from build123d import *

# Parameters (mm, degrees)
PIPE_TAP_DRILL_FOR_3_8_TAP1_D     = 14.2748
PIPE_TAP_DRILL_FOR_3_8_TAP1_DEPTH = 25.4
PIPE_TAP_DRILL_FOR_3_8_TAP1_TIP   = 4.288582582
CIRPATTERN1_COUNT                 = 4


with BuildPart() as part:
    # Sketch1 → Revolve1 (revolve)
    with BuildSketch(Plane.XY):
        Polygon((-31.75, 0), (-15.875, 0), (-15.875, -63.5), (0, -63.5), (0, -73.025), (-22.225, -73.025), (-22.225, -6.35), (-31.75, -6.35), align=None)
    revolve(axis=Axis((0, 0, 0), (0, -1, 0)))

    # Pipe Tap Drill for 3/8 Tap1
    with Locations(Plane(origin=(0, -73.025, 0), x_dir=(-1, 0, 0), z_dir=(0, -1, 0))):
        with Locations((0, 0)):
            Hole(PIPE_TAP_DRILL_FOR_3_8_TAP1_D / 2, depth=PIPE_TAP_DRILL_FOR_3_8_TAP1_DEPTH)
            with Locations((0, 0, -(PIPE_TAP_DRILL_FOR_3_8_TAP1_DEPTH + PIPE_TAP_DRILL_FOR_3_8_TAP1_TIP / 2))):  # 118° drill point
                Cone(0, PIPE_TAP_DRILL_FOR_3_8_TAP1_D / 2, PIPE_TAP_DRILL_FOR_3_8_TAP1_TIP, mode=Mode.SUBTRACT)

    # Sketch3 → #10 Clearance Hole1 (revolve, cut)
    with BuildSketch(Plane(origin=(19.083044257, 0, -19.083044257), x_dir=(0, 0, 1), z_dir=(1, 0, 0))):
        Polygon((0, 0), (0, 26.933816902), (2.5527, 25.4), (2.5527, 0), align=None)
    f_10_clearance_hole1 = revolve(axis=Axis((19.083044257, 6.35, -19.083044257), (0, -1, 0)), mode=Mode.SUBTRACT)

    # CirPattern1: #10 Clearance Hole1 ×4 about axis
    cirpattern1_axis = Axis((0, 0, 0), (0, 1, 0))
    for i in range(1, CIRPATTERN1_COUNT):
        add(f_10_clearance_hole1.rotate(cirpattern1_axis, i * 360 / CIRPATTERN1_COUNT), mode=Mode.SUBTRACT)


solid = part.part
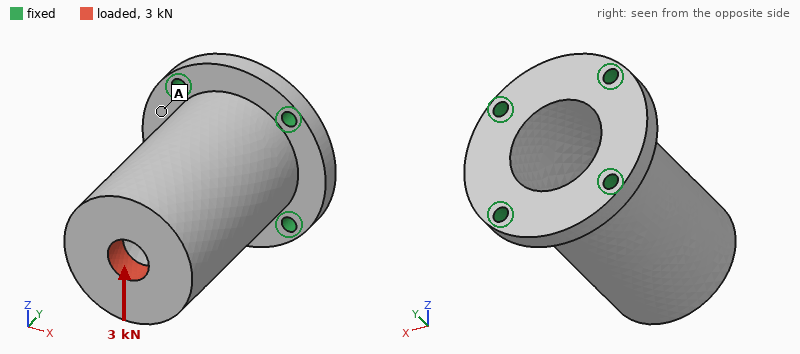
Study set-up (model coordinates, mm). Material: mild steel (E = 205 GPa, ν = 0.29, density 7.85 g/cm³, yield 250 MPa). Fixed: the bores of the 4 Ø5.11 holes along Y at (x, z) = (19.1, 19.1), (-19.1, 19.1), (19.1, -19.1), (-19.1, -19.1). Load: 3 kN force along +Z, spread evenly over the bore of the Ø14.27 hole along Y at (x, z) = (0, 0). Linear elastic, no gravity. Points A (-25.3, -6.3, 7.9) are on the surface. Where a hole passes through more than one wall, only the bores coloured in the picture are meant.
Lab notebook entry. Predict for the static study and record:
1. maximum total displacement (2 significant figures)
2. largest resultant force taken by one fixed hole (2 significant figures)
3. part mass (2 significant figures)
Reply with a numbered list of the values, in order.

1. 34 µm
2. 2.9 kN
3. 560 g
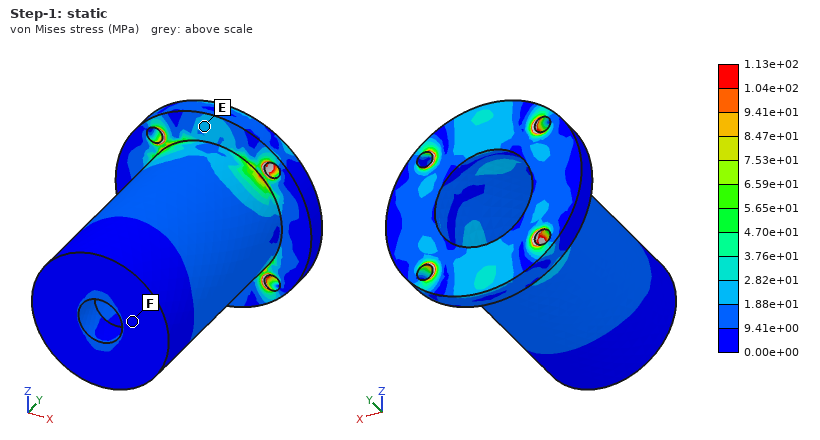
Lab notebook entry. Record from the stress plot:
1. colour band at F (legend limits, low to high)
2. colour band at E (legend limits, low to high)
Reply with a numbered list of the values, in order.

1. 0.00e+00 to 9.41e+00 MPa
2. 1.88e+01 to 2.82e+01 MPa
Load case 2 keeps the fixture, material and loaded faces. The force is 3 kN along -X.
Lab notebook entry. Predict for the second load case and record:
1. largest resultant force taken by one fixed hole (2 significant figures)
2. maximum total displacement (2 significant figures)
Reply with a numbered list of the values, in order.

1. 2.9 kN
2. 34 µm
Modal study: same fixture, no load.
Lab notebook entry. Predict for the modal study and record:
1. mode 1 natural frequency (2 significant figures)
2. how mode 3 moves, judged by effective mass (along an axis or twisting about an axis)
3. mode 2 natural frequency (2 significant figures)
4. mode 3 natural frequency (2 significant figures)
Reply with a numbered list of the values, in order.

1. 3500 Hz
2. along Y
3. 3500 Hz
4. 9900 Hz
